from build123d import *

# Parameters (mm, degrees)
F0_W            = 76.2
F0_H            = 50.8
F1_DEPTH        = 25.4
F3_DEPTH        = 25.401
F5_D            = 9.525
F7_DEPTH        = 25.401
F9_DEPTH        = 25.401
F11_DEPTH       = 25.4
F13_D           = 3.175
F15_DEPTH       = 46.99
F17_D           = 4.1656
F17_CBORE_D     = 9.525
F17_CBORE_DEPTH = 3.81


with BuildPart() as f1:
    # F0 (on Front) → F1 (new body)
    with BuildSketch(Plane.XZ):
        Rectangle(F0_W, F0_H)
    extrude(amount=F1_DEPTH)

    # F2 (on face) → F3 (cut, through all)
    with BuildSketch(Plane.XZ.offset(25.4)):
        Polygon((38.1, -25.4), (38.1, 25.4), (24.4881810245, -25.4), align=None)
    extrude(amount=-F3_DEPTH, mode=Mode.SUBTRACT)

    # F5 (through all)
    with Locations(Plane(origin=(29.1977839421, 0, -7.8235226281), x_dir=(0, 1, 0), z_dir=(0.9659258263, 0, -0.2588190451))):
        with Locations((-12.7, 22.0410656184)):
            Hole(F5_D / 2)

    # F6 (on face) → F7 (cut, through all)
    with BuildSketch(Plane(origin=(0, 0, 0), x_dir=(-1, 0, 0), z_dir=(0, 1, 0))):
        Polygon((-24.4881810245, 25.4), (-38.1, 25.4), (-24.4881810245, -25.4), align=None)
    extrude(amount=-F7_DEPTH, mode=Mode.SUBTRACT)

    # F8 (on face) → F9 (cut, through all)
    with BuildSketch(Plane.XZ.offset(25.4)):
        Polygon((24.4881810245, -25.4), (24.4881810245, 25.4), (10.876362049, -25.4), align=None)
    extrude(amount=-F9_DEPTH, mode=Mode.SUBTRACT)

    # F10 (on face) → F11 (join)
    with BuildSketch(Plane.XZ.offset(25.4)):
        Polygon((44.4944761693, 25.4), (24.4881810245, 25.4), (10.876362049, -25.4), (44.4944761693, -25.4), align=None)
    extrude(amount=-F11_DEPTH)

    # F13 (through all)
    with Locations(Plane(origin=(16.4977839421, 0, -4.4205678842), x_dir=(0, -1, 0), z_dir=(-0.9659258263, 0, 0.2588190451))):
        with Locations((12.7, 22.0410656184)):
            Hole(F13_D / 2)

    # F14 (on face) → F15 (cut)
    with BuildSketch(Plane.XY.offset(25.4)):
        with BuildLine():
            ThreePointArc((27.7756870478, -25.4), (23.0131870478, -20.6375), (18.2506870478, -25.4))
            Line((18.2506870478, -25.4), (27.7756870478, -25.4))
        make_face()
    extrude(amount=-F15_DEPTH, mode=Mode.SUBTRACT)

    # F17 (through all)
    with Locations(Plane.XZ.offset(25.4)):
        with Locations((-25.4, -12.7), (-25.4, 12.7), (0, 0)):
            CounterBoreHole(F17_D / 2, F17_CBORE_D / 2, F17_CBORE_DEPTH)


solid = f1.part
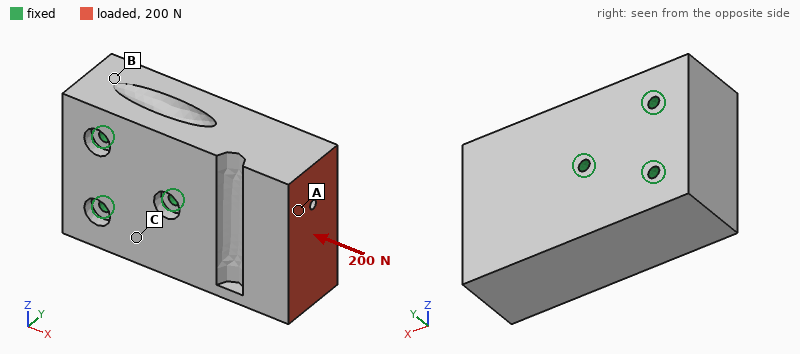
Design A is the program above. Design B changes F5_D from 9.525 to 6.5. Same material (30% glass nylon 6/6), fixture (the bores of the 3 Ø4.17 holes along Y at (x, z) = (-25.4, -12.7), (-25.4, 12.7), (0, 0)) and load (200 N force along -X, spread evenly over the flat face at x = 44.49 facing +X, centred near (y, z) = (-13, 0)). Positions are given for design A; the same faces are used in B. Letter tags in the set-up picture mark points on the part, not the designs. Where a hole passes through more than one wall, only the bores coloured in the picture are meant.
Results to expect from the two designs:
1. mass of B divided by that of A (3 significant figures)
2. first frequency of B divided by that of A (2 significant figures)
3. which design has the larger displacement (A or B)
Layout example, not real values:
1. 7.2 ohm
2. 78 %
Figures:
1. 1.01
2. 1.0
3. A
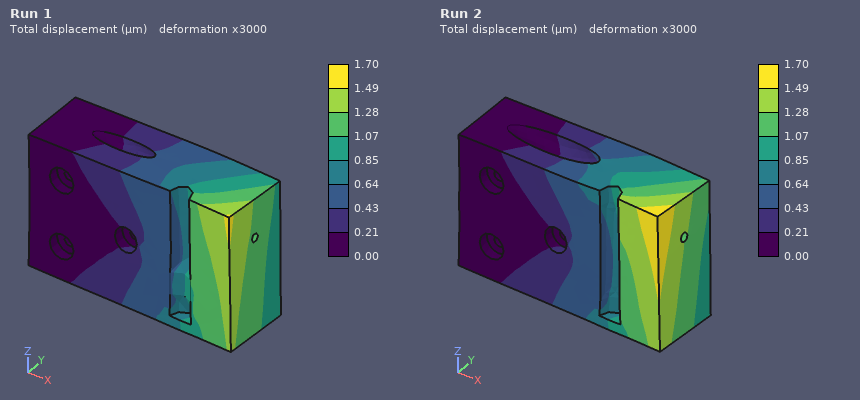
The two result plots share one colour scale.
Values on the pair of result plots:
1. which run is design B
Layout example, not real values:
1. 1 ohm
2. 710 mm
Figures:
1. Run 1
